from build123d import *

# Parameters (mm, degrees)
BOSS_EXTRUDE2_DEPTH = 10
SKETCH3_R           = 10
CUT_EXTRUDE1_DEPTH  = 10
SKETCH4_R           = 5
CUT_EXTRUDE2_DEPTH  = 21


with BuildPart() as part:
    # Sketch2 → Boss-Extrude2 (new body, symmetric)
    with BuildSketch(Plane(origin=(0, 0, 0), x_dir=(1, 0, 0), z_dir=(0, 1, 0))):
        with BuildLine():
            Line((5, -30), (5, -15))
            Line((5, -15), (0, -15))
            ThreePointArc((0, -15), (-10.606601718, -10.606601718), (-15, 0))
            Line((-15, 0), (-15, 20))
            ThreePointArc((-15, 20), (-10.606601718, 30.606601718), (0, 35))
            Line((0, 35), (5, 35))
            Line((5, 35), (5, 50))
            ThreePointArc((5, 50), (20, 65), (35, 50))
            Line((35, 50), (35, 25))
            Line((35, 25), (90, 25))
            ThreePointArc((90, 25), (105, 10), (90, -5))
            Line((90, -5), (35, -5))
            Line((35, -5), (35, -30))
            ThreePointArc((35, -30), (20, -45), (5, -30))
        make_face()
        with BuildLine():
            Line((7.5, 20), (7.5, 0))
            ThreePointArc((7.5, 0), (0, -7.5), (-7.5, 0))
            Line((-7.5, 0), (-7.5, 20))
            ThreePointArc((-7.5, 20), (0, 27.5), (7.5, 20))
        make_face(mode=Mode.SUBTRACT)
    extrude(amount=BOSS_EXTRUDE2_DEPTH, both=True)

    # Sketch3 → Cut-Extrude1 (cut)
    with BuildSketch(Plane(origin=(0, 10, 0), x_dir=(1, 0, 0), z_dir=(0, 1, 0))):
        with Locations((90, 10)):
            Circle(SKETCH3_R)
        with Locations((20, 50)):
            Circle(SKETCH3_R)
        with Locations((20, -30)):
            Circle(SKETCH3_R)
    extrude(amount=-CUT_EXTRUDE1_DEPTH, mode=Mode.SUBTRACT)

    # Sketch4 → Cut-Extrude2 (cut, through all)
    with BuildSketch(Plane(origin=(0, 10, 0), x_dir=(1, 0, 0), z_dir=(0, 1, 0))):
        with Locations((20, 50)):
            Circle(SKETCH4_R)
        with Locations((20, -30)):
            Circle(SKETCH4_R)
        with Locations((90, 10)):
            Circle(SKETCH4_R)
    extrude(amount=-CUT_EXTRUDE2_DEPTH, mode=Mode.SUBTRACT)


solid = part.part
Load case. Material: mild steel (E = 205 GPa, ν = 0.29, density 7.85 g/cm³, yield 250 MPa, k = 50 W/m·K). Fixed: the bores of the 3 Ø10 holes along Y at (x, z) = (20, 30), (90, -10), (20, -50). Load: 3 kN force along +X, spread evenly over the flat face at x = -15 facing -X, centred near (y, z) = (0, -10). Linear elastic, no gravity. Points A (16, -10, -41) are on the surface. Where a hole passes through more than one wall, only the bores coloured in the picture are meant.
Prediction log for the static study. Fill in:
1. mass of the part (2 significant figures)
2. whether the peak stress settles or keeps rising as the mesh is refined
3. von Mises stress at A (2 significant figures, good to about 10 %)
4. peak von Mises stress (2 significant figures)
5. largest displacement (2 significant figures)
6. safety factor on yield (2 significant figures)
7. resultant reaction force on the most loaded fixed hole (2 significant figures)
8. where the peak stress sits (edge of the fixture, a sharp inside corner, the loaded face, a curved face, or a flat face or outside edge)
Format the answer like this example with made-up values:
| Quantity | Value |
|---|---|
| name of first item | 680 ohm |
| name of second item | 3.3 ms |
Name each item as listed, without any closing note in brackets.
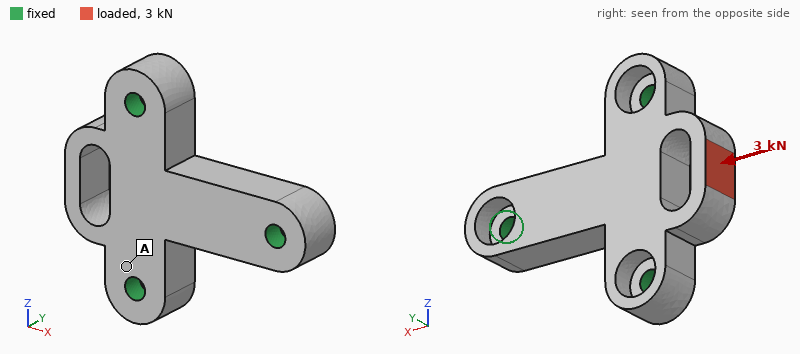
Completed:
| Quantity | Value |
|---|---|
| mass of the part | 780 g |
| whether the peak stress settles or keeps rising as the mesh is refined | settles |
| von Mises stress at A | 6.1 MPa |
| peak von Mises stress | 58 MPa |
| largest displacement | 10 µm |
| safety factor on yield | 4.3 |
| resultant reaction force on the most loaded fixed hole | 1.3 kN |
| where the peak stress sits | a curved face |
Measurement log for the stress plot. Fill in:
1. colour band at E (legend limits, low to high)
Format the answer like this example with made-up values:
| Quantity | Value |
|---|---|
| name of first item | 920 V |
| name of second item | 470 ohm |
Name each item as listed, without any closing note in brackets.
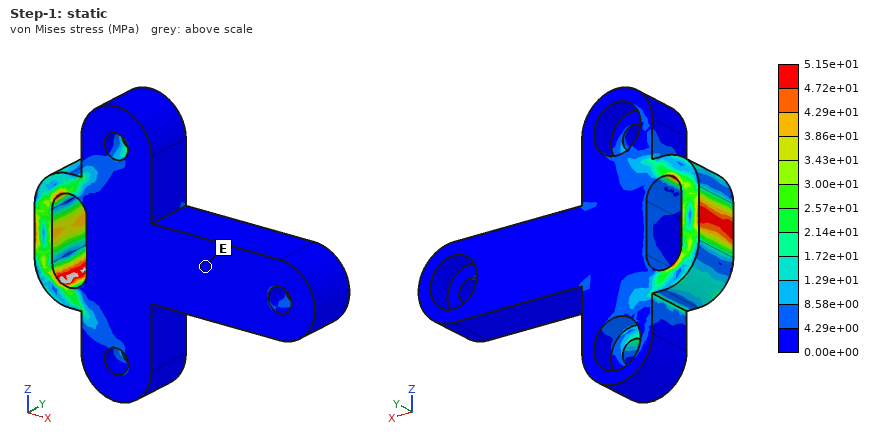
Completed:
| Quantity | Value |
|---|---|
| colour band at E | 0.00e+00 to 4.29e+00 MPa |
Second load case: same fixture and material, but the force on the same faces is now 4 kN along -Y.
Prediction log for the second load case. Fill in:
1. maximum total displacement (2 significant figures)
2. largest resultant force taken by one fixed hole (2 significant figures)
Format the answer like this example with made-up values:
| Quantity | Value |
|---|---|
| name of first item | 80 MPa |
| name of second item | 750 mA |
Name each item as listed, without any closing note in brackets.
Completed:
| Quantity | Value |
|---|---|
| maximum total displacement | 48 µm |
| largest resultant force taken by one fixed hole | 3.3 kN |
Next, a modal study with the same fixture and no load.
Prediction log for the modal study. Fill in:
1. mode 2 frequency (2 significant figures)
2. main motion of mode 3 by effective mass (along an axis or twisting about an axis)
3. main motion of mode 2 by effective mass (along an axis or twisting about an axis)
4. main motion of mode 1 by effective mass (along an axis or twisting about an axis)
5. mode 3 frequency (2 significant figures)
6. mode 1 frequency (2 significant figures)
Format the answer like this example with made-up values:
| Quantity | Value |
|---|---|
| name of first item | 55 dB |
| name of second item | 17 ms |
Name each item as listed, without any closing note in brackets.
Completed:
| Quantity | Value |
|---|---|
| mode 2 frequency | 9100 Hz |
| main motion of mode 3 by effective mass | along Z |
| main motion of mode 2 by effective mass | along Y |
| main motion of mode 1 by effective mass | along Y |
| mode 3 frequency | 12 kHz |
| mode 1 frequency | 6800 Hz |
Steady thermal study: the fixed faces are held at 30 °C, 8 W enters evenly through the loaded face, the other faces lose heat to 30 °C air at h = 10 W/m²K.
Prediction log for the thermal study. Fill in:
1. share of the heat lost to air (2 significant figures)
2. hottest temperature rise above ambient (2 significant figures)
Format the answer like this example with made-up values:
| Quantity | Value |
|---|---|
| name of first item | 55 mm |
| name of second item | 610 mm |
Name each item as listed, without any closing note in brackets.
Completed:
| Quantity | Value |
|---|---|
| share of the heat lost to air | 7.8 % |
| hottest temperature rise above ambient | 20 K |
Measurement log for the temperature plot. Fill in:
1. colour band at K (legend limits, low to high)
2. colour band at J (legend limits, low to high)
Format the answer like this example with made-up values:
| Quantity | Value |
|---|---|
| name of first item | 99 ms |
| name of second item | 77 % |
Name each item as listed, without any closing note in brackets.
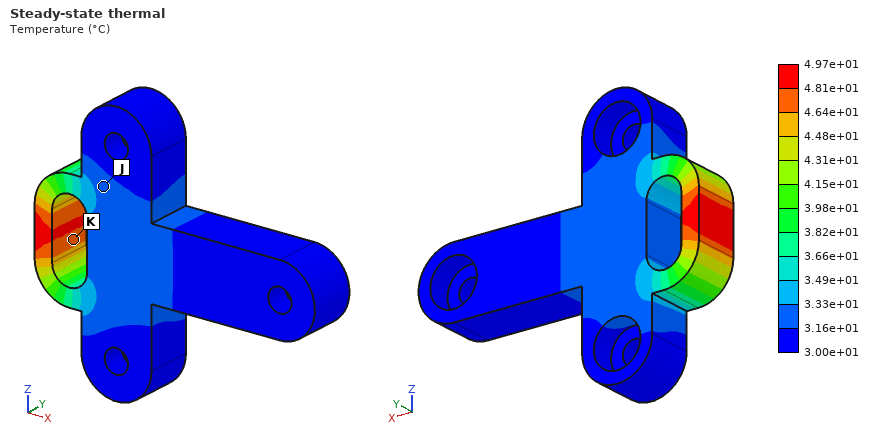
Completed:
| Quantity | Value |
|---|---|
| colour band at K | 4.64e+01 to 4.81e+01 °C |
| colour band at J | 3.16e+01 to 3.33e+01 °C |
